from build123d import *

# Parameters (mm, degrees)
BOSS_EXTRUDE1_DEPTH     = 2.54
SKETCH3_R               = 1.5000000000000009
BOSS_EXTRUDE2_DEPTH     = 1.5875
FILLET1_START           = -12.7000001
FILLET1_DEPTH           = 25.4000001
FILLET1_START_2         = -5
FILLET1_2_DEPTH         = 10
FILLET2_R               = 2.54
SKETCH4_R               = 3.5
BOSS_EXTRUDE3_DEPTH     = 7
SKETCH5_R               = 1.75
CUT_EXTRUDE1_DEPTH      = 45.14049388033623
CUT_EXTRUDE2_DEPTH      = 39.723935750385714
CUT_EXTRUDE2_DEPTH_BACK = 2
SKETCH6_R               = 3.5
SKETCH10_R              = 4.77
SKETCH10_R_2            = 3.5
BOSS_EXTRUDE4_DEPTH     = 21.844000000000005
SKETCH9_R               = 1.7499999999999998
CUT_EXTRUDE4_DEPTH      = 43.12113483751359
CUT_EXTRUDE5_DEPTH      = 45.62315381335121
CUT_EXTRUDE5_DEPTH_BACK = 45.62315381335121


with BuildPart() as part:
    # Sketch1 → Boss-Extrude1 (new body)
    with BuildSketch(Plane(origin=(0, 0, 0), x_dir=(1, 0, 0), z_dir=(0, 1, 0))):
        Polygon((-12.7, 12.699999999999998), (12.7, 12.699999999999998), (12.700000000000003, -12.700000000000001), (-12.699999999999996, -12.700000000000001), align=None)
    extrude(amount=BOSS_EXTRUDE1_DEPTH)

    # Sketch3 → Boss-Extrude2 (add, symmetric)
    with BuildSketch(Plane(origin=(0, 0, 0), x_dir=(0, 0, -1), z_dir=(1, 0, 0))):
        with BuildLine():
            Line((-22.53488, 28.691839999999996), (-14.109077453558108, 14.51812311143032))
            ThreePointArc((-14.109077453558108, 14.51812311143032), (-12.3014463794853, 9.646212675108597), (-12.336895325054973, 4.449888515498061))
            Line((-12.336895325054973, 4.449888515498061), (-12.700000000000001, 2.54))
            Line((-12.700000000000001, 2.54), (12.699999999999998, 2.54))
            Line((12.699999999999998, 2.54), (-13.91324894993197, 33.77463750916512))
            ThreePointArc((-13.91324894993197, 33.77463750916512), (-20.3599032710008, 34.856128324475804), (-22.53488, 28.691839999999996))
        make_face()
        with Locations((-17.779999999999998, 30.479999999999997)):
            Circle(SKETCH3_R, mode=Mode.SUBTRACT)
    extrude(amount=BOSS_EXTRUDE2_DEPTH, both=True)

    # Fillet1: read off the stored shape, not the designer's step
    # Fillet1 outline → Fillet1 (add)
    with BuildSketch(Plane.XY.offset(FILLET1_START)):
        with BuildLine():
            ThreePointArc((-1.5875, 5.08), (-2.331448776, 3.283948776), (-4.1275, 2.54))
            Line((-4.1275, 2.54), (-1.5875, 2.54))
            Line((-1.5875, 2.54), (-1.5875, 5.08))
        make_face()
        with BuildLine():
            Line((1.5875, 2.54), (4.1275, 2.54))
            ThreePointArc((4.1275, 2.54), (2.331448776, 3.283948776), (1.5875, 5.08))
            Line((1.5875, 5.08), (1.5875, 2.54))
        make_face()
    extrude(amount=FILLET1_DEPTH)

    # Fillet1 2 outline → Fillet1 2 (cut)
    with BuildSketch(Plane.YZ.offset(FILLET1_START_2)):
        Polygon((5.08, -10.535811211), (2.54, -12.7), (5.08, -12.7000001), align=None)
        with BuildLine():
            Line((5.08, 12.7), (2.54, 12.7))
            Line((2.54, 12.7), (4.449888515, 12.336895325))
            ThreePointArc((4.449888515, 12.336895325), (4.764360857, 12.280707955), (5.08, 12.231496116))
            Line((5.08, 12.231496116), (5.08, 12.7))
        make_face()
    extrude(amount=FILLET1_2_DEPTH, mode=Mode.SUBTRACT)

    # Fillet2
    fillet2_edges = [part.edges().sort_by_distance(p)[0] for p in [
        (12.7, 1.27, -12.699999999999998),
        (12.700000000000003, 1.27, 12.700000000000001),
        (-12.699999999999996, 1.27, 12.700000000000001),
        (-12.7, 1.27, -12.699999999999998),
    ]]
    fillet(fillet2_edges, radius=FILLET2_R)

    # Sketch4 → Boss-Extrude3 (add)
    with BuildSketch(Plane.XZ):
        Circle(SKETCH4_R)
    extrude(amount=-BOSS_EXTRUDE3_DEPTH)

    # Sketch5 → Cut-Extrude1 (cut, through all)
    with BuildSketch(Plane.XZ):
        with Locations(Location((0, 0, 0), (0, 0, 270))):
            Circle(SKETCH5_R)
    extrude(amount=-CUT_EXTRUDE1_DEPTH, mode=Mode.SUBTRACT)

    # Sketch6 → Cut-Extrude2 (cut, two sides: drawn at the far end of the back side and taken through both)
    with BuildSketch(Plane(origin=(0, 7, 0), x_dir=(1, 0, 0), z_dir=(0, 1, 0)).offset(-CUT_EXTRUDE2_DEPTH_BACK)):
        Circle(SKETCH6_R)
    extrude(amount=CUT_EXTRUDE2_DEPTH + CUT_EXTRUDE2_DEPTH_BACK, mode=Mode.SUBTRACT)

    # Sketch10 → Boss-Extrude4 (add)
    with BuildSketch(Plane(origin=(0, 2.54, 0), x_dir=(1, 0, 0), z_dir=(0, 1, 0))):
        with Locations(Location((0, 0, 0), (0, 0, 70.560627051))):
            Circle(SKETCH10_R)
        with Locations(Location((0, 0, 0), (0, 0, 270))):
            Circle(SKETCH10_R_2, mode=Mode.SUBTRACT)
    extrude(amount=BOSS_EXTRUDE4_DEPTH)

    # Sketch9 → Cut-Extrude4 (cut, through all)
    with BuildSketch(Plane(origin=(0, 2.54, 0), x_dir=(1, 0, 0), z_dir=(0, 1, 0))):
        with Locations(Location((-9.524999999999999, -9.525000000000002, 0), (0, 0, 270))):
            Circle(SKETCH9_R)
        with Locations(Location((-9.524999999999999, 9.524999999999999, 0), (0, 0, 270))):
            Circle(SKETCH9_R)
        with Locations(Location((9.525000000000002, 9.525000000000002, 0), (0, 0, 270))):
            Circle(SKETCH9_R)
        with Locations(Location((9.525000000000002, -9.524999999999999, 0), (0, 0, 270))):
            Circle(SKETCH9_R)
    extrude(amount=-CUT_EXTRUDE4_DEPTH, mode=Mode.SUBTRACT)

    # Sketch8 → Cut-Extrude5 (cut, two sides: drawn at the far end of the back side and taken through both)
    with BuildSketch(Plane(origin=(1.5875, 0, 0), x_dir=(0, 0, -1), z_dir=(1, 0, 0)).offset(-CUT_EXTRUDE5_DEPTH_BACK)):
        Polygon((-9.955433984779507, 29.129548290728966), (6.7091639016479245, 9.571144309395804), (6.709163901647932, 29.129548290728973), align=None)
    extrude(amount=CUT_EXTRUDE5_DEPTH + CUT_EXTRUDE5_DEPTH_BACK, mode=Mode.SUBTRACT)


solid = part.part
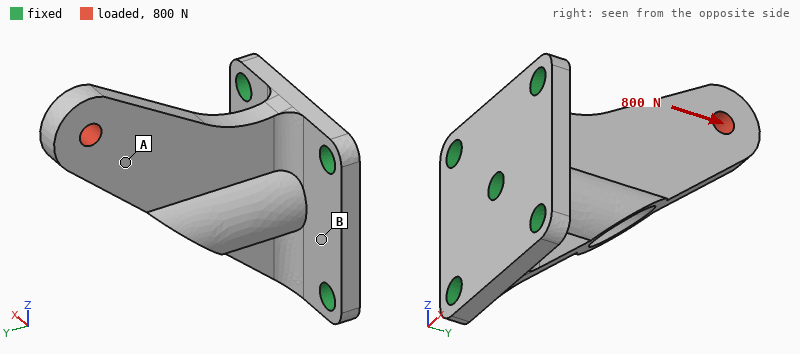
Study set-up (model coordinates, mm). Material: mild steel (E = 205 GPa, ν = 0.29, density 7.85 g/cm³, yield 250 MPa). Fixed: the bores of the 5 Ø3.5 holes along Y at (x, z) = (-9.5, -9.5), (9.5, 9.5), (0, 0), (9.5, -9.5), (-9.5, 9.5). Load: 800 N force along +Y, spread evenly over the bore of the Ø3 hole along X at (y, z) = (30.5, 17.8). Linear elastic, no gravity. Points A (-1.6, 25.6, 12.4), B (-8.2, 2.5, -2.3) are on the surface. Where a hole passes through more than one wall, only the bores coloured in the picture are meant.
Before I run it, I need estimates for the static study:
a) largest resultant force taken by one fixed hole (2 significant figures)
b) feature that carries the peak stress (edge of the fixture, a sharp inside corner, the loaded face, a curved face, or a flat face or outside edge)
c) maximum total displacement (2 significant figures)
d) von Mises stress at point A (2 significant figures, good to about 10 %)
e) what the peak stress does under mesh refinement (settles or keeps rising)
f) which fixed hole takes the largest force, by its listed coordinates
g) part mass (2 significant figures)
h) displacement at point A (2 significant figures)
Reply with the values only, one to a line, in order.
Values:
460 N
edge of the fixture
59 µm
29 MPa
keeps rising
(0, 0)
26 g
33 µm
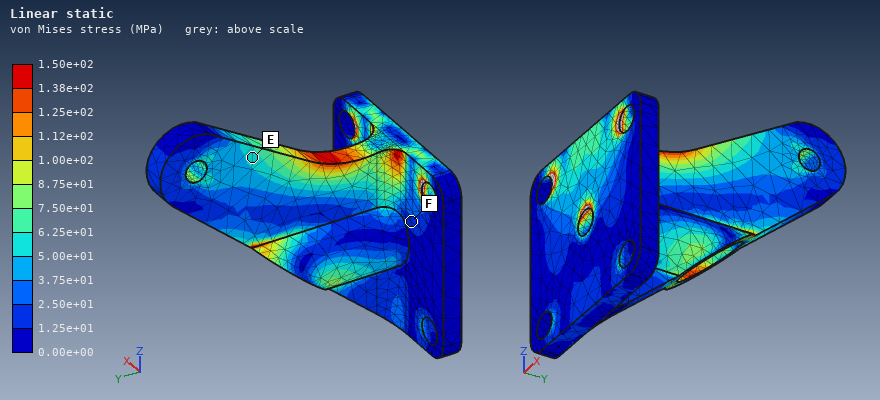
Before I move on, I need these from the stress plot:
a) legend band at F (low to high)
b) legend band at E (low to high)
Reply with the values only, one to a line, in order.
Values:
1.25e+01 to 2.50e+01 MPa
5.00e+01 to 6.25e+01 MPa
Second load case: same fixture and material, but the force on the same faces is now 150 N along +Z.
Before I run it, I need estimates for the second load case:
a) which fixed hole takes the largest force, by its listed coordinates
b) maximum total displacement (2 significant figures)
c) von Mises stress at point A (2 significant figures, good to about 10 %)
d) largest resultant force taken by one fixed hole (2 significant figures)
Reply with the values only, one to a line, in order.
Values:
(0, 0)
18 µm
9.5 MPa
240 N
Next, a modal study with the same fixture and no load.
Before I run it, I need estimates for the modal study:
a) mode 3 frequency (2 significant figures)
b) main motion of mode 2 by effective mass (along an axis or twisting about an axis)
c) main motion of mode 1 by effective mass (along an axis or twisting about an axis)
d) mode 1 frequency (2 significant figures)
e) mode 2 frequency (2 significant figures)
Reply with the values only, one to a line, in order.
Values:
14 kHz
along Z
along X
3900 Hz
7900 Hz
